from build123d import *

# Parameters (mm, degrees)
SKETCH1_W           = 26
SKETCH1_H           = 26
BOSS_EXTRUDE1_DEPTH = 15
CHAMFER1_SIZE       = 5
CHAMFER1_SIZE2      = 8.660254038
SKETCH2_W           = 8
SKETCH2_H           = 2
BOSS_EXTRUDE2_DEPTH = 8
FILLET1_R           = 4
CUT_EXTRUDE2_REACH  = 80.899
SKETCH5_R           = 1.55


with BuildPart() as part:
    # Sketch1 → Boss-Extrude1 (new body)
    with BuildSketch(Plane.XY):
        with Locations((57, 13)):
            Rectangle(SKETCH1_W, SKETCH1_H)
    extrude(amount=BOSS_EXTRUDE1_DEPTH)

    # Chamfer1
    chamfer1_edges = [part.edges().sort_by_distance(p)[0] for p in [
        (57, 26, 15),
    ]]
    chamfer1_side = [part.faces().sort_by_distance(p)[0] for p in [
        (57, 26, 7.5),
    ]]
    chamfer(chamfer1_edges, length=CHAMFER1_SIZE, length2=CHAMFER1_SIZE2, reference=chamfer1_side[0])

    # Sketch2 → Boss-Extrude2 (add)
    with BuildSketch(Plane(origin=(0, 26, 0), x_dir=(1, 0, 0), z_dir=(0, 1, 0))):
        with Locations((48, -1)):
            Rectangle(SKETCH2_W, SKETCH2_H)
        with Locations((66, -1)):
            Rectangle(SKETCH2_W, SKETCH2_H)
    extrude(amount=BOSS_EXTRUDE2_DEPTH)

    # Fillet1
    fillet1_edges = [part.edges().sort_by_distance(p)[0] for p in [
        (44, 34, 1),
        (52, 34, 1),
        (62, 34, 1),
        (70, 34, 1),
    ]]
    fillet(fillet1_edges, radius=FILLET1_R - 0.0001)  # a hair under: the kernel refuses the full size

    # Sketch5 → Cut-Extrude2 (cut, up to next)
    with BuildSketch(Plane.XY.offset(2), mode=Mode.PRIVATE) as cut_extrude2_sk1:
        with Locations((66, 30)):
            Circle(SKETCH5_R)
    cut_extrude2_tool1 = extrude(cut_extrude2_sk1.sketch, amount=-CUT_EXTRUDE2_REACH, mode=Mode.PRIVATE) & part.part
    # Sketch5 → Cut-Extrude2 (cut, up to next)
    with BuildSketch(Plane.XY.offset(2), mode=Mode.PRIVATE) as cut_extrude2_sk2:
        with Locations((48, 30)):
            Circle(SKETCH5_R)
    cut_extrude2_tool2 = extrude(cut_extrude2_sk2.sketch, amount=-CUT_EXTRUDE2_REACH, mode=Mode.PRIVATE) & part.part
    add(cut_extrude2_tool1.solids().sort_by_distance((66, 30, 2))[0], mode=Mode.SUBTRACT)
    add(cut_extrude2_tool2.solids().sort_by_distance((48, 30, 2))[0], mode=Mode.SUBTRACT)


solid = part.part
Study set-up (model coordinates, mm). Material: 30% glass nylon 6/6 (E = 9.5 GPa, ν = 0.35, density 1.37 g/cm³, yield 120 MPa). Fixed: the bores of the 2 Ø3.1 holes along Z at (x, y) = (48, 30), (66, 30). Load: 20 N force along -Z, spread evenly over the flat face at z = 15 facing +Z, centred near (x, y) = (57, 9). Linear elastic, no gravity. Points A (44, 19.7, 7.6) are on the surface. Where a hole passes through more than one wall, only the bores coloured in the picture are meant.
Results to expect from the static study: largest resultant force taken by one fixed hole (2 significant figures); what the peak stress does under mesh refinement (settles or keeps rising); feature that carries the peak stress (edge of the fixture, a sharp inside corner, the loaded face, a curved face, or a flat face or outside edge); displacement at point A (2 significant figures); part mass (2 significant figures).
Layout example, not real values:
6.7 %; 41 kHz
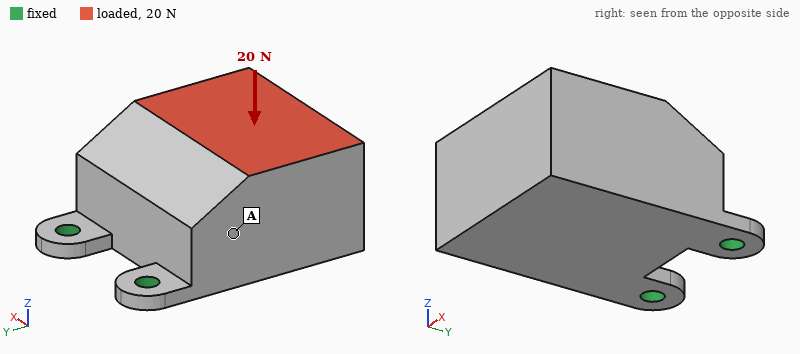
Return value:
10 N; keeps rising; edge of the fixture; 0.14 mm; 13 g
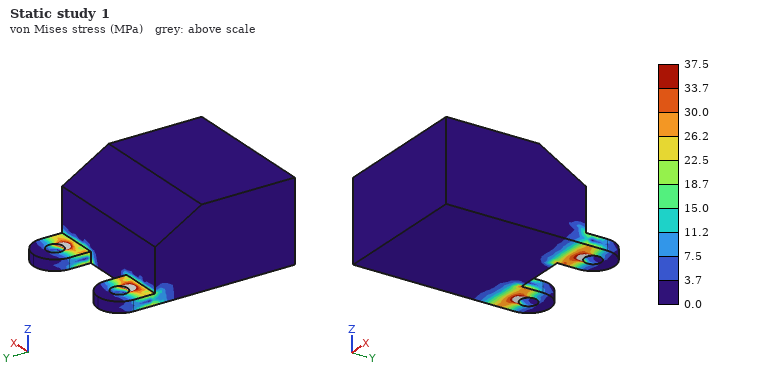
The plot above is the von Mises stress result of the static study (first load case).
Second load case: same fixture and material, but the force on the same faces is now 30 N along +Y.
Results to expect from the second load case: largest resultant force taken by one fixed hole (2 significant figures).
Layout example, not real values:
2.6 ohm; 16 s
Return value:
15 N
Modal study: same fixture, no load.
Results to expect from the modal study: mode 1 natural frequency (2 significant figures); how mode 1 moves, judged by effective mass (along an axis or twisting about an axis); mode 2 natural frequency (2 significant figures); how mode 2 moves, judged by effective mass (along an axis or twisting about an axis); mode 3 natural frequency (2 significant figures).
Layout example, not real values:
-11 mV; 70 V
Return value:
390 Hz; along Z; 3100 Hz; along X; 4300 Hz
